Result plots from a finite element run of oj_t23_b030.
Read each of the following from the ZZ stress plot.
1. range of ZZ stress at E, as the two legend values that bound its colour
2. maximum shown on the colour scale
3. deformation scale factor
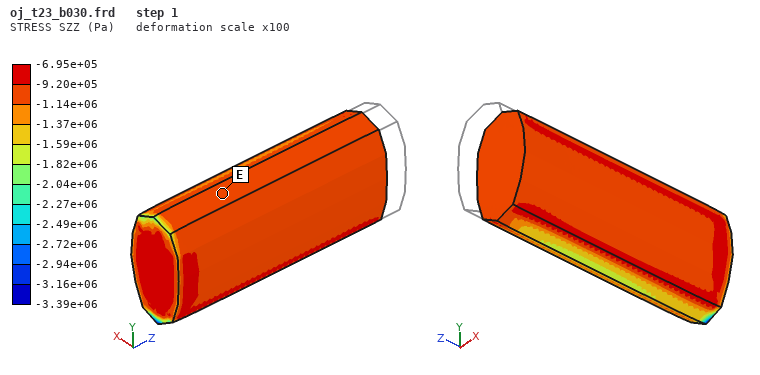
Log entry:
-1.14e+06 to -9.20e+05 Pa
-6.95e+05 Pa
100
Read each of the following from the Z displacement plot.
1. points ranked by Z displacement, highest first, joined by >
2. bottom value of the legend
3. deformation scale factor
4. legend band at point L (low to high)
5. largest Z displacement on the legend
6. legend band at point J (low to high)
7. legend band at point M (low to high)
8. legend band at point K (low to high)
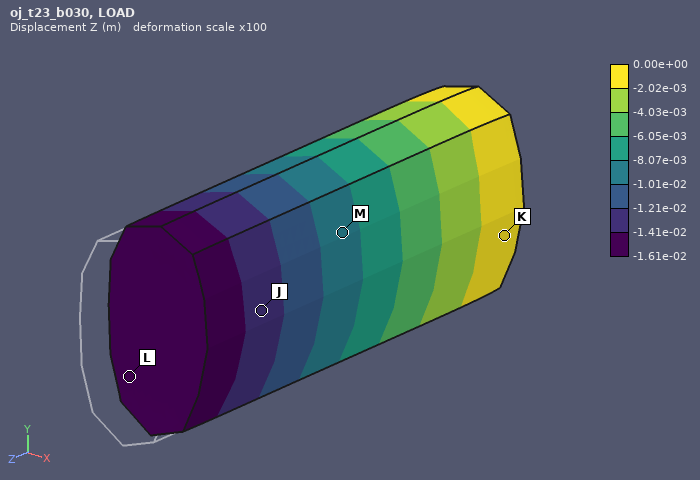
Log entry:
K > M > J > L
-1.61e-02 m
100
-1.61e-02 to -1.41e-02 m
0.00e+00 m
-1.41e-02 to -1.21e-02 m
-1.01e-02 to -8.07e-03 m
-2.02e-03 to 0.00e+00 m
